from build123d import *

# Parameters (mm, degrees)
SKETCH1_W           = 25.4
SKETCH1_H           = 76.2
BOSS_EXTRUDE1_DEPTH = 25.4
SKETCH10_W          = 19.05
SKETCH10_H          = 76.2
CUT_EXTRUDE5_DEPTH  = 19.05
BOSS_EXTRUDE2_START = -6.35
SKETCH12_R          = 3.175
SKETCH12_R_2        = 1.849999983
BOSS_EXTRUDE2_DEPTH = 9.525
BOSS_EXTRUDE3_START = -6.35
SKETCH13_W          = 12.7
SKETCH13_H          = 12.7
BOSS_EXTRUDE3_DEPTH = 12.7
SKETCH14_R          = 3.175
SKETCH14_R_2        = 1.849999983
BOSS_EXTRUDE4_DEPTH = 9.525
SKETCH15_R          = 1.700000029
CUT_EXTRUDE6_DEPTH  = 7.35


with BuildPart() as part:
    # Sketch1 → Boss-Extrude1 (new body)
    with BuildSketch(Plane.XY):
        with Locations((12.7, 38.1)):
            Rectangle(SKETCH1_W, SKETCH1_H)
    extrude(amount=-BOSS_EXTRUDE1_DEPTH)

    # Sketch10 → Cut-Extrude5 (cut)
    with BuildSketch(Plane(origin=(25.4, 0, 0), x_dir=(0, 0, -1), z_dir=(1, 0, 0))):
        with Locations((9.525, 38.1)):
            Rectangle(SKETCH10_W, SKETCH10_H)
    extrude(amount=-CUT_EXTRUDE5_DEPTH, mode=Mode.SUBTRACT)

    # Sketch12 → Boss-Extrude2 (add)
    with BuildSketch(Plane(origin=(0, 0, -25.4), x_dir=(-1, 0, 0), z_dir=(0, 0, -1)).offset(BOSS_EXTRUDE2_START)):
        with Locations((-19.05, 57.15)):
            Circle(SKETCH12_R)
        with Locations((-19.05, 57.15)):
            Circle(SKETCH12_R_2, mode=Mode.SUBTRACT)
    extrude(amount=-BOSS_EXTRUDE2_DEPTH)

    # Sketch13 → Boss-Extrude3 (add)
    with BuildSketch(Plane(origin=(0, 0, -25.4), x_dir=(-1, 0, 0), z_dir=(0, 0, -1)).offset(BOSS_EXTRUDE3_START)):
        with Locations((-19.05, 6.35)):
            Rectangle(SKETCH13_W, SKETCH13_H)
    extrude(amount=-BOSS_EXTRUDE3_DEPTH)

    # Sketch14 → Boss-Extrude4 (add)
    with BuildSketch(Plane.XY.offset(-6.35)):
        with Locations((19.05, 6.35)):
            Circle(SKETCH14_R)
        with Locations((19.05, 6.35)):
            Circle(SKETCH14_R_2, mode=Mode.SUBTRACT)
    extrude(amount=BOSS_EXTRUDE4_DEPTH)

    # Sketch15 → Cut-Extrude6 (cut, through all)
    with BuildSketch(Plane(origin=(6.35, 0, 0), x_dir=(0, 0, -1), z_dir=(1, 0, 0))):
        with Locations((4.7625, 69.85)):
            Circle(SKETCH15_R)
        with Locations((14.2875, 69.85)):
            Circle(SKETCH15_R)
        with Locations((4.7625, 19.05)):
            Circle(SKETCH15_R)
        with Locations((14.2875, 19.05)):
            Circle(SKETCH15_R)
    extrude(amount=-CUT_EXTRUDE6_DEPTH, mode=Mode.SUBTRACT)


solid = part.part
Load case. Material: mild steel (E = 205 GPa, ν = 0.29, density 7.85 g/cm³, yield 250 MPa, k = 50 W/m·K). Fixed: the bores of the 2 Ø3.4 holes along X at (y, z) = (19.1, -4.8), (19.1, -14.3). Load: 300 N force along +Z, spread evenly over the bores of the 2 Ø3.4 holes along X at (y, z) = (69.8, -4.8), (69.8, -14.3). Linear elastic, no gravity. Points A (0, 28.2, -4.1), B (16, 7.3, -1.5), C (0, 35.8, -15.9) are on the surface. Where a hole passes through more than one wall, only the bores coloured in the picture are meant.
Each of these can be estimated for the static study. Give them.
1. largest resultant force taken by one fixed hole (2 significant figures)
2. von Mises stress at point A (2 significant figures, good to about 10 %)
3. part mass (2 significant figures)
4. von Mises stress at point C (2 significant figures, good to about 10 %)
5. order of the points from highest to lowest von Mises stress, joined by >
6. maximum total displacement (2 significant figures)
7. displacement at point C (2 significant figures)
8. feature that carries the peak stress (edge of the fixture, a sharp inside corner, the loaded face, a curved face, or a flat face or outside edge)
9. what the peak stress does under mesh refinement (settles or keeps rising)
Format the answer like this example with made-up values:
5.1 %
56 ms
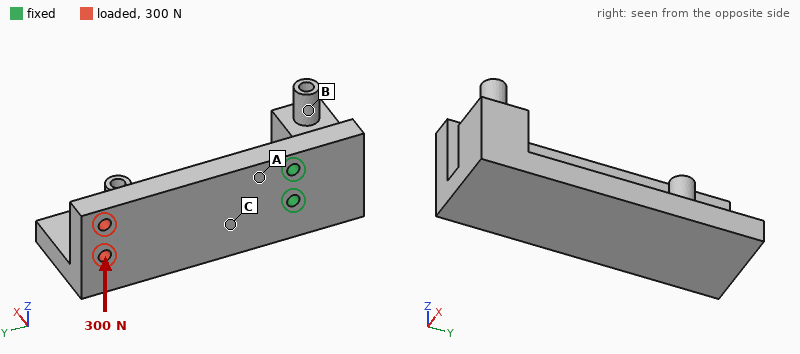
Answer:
1.3 kN
13 MPa
190 g
6.1 MPa
A > C > B
13 µm
2.7 µm
edge of the fixture
keeps rising
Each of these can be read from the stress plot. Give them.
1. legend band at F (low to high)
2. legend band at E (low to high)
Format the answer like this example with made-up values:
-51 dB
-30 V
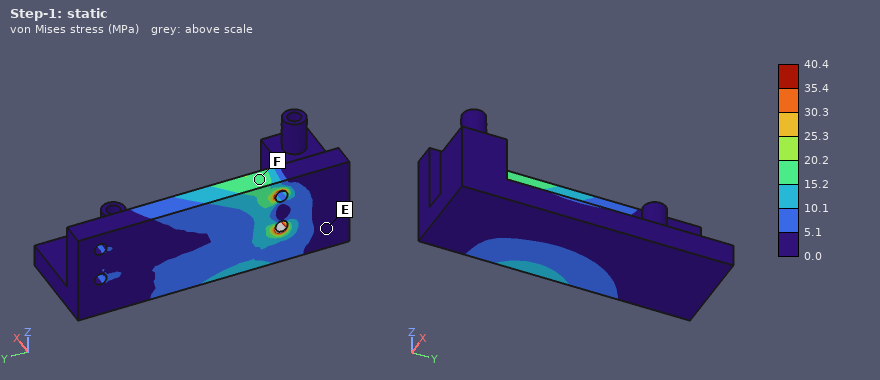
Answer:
15.2 to 20.2 MPa
0.0 to 5.1 MPa
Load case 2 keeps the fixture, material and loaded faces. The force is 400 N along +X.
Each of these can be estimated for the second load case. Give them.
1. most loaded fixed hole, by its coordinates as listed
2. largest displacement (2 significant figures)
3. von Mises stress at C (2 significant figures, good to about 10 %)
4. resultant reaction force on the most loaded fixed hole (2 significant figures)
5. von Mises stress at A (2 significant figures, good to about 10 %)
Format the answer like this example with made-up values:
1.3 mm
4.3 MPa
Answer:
(19.1, -14.3)
68 µm
18 MPa
220 N
37 MPa
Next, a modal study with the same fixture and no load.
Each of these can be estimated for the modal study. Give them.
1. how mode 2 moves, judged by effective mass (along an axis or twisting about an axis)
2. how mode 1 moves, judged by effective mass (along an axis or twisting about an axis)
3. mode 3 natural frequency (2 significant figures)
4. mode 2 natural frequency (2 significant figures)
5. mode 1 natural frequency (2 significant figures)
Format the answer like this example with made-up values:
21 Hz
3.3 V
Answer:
along Z
along X
4200 Hz
3200 Hz
1800 Hz
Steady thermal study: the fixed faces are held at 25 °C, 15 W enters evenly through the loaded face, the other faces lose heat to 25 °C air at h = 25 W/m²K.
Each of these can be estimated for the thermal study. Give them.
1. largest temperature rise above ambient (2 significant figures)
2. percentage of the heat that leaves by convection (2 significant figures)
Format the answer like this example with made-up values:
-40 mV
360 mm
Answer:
64 K
32 %
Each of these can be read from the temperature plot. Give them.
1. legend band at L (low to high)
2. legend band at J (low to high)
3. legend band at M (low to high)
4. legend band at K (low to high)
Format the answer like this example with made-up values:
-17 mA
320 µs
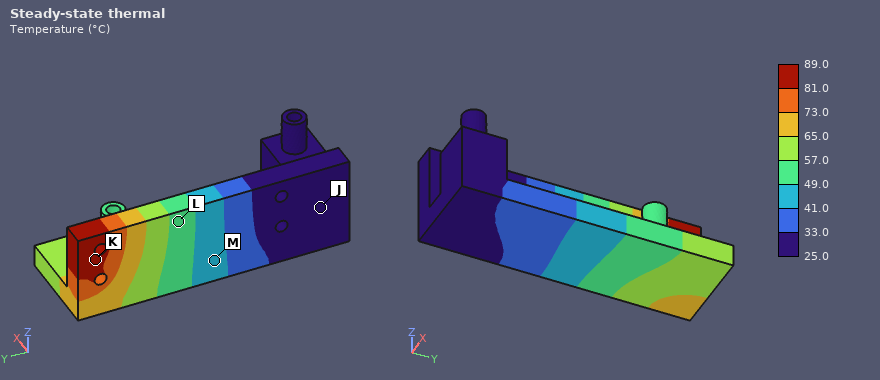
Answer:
49.0 to 57.0 °C
25.0 to 33.0 °C
41.0 to 49.0 °C
81.0 to 89.0 °C
